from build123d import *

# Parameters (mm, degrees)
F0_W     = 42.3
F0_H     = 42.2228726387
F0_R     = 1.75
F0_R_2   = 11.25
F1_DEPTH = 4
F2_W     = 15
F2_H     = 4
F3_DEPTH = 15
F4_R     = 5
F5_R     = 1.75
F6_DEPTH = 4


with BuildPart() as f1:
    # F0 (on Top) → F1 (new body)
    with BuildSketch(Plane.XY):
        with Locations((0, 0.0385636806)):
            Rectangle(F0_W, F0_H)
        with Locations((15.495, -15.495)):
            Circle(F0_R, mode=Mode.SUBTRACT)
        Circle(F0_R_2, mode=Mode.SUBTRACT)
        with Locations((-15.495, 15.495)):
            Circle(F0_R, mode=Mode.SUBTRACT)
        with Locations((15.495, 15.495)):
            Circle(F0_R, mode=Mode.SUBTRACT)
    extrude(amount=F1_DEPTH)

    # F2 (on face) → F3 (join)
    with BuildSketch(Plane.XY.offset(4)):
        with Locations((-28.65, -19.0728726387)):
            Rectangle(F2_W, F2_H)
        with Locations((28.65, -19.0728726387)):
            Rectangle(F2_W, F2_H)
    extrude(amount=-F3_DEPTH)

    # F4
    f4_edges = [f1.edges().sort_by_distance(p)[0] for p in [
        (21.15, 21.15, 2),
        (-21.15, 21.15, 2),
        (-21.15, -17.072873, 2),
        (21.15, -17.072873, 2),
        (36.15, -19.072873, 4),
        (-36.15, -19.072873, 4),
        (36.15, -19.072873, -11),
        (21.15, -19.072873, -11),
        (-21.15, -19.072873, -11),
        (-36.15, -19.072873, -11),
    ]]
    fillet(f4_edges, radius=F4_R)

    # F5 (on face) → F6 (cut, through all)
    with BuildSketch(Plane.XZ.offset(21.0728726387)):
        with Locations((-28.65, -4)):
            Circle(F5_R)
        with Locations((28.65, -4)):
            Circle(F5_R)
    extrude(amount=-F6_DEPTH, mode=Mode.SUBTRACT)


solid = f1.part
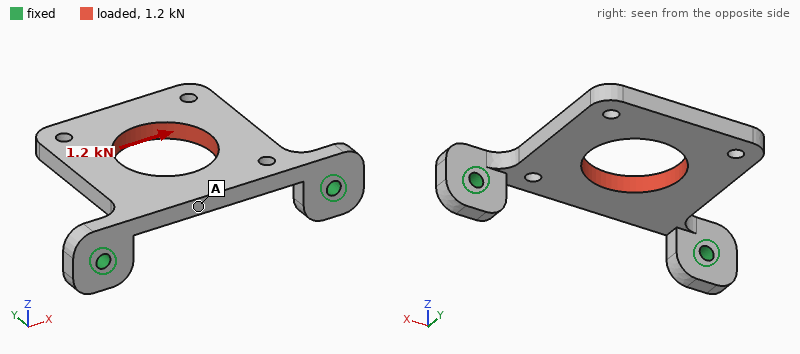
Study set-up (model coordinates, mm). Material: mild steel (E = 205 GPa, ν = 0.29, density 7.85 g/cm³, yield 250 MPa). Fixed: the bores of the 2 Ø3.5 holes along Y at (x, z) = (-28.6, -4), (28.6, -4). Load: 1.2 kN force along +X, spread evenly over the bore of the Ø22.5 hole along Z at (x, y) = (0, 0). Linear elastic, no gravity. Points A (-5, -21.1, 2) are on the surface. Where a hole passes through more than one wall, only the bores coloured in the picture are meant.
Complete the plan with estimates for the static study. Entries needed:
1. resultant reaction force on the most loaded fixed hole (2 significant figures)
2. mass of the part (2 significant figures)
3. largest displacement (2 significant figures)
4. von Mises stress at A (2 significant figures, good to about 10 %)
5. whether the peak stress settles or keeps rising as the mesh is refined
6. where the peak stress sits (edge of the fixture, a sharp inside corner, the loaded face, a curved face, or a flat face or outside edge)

760 N
55 g
23 µm
16 MPa
keeps rising
edge of the fixture
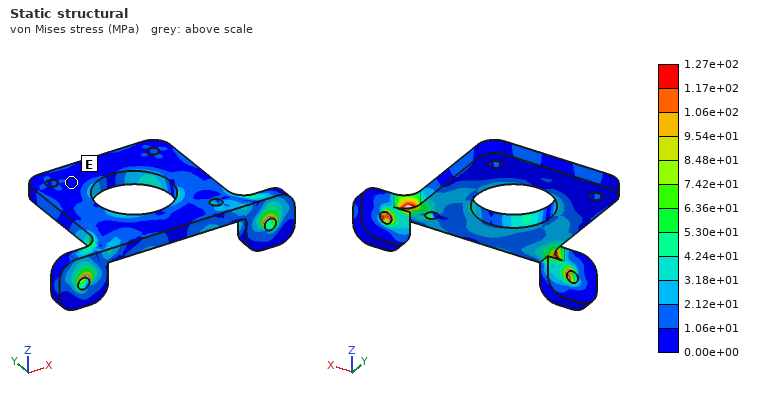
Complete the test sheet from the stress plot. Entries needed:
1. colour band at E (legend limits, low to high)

0.00e+00 to 1.06e+01 MPa
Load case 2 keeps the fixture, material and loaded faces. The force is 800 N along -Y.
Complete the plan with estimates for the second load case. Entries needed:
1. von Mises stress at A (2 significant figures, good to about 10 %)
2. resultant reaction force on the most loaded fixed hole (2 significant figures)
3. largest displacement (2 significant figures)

14 MPa
440 N
36 µm
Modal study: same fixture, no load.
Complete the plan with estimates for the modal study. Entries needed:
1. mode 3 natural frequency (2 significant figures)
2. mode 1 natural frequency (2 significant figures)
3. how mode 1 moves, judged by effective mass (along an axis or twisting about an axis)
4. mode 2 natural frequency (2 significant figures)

6600 Hz
1100 Hz
along Z
3600 Hz
